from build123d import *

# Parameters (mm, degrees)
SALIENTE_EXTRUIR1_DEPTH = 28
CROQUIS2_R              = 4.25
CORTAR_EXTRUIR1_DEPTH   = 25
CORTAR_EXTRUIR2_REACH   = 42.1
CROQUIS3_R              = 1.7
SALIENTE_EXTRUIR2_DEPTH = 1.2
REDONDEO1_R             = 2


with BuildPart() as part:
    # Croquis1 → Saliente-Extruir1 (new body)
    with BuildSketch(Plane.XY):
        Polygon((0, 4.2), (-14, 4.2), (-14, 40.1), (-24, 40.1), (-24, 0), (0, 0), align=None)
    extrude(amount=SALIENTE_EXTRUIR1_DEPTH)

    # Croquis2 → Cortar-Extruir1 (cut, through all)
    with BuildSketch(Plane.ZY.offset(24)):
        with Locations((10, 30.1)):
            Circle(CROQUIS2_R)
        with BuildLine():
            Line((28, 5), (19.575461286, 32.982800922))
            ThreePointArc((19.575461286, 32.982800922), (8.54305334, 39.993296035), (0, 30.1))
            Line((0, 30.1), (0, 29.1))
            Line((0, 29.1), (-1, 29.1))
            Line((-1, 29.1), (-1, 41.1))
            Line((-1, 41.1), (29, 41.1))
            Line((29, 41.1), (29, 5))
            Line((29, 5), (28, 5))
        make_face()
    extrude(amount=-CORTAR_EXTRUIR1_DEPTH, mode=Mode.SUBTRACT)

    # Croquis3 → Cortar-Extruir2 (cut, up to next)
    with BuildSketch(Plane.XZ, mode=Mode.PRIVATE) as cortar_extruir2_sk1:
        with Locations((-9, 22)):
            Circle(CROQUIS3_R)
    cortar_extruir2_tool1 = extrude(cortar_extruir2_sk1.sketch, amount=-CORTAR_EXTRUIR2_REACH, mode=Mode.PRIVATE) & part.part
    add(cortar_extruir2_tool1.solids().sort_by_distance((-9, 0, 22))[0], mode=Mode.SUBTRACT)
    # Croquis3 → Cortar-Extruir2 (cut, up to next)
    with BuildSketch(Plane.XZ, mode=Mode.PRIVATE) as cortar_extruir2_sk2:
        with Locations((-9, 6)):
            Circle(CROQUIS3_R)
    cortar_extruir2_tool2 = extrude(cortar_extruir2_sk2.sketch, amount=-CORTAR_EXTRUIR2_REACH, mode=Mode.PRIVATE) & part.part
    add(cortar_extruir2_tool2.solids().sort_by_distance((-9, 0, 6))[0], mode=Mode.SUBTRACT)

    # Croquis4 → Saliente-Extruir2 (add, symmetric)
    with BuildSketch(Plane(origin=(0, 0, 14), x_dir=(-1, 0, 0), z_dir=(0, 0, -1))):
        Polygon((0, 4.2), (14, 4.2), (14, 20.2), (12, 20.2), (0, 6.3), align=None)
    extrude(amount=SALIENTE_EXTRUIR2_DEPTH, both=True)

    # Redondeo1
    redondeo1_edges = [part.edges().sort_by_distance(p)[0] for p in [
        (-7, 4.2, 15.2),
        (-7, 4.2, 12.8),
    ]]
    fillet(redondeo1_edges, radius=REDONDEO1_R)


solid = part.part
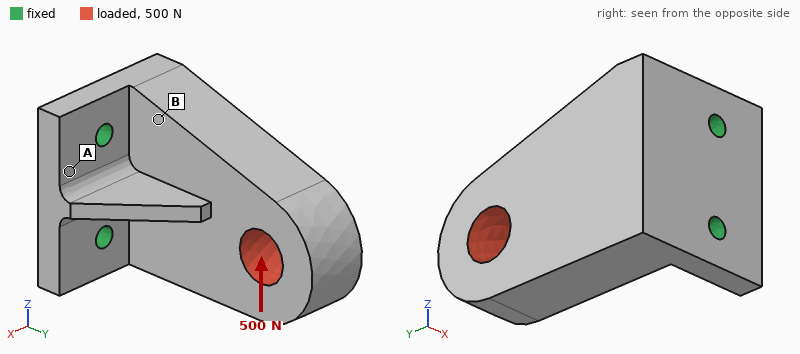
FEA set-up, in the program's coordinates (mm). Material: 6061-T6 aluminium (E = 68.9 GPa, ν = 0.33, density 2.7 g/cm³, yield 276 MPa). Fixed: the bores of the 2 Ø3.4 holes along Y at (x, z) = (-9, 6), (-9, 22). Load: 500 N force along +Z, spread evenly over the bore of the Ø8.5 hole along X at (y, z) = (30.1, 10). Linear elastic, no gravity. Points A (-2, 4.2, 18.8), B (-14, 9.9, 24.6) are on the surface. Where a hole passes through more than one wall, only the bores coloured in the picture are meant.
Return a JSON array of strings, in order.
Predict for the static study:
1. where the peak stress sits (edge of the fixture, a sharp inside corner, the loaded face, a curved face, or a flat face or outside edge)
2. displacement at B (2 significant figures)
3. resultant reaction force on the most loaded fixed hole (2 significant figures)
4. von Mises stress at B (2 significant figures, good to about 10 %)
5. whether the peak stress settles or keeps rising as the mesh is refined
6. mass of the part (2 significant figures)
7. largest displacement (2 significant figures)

["edge of the fixture", "15 µm", "850 N", "19 MPa", "keeps rising", "28 g", "49 µm"]
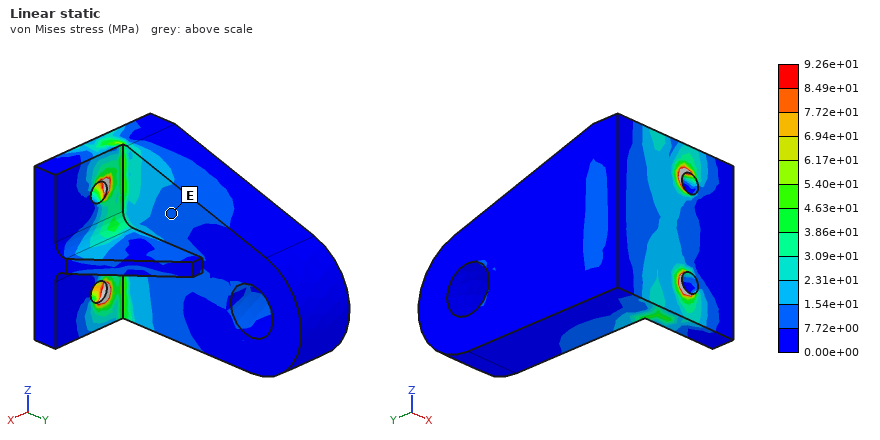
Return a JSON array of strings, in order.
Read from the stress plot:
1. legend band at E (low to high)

["7.72e+00 to 1.54e+01 MPa"]
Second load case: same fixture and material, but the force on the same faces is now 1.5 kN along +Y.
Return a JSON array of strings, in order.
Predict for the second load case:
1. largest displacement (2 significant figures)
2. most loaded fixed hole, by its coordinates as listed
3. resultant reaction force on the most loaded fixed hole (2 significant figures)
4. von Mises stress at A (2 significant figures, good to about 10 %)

["0.14 mm", "(-9, 6)", "1.1 kN", "26 MPa"]
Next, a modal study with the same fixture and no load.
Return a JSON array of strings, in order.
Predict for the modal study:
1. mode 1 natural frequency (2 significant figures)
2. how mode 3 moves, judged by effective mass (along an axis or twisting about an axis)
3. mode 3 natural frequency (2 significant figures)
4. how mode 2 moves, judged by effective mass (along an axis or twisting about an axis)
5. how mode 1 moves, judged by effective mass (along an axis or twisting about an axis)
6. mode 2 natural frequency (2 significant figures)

["3100 Hz", "along Y", "14 kHz", "along Z", "along X", "5700 Hz"]
